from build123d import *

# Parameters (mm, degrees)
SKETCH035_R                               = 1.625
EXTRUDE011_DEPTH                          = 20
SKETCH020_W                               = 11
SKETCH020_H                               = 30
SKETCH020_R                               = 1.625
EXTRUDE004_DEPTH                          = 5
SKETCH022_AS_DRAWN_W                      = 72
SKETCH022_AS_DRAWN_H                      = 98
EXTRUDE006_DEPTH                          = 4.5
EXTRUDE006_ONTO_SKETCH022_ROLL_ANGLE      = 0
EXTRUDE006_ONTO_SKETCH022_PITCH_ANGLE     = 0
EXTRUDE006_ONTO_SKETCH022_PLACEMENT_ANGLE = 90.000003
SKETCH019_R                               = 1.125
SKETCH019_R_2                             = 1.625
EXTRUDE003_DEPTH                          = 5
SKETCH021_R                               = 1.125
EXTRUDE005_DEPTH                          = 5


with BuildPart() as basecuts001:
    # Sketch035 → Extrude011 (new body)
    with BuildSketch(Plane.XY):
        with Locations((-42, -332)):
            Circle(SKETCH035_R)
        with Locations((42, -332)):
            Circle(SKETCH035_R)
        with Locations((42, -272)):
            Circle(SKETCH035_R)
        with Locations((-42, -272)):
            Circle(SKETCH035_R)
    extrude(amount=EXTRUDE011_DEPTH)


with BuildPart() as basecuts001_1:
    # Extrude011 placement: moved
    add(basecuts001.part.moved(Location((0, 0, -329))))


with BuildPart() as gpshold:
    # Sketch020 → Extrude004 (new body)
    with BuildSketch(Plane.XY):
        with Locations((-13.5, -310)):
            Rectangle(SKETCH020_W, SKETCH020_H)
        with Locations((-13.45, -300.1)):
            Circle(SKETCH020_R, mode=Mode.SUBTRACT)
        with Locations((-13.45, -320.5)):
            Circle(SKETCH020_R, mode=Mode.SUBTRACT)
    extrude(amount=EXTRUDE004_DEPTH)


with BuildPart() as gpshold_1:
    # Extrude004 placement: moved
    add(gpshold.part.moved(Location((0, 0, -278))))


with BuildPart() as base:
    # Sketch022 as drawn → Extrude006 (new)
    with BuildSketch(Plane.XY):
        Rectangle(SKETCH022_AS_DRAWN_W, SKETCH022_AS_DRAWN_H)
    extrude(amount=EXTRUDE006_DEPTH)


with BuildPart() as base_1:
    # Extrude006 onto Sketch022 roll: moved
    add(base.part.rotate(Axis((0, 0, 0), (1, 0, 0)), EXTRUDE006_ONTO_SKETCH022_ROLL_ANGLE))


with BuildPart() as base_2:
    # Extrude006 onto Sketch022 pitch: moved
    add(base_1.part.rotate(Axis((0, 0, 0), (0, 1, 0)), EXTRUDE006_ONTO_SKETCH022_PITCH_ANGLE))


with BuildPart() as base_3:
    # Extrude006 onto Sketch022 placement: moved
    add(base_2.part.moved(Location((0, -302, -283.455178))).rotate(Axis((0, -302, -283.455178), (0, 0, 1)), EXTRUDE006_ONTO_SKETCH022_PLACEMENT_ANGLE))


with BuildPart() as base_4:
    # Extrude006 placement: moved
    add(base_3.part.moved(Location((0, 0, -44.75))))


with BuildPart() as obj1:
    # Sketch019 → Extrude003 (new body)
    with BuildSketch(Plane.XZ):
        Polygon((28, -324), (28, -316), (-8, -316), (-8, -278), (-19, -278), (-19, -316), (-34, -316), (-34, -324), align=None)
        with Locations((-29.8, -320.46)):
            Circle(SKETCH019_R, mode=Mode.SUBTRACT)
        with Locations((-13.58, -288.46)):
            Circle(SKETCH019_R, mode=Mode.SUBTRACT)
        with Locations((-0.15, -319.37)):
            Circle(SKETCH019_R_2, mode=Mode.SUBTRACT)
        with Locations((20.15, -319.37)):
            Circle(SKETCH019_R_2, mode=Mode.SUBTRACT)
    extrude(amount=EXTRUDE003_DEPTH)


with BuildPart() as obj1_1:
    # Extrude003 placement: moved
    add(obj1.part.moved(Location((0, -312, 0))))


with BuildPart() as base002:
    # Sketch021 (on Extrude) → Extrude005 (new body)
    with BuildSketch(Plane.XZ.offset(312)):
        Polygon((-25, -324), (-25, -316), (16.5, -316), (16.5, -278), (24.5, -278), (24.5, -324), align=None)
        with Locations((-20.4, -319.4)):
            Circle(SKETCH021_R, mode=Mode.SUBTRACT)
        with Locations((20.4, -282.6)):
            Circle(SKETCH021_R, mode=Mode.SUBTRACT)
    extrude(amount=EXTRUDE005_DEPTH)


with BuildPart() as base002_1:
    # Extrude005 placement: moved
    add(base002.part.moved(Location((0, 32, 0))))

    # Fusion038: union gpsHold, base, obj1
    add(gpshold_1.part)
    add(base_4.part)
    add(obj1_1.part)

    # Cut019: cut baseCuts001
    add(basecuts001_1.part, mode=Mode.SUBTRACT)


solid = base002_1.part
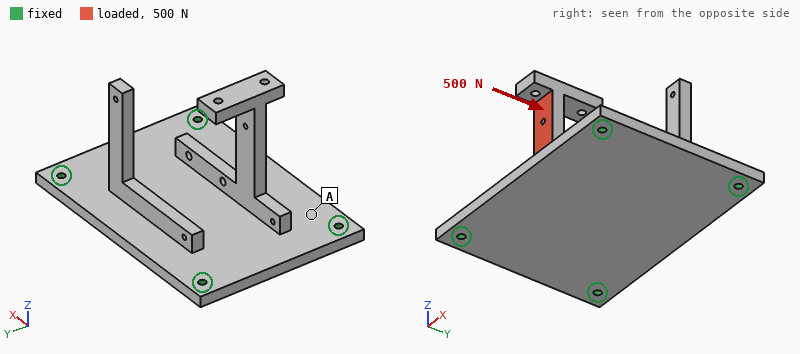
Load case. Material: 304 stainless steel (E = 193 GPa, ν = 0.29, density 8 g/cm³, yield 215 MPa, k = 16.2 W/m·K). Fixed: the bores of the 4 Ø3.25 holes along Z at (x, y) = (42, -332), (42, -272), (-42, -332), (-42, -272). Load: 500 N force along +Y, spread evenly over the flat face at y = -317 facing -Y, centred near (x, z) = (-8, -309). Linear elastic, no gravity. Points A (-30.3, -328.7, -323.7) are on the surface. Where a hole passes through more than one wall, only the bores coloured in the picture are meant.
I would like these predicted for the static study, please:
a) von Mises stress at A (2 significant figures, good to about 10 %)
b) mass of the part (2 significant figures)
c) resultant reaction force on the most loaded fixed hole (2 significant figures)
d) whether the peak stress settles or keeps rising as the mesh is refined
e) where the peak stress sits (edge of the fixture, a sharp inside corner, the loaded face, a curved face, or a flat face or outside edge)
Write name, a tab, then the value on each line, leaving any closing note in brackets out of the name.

von Mises stress at A	11 MPa
mass of the part	330 g
resultant reaction force on the most loaded fixed hole	210 N
whether the peak stress settles or keeps rising as the mesh is refined	keeps rising
where the peak stress sits	a sharp inside corner
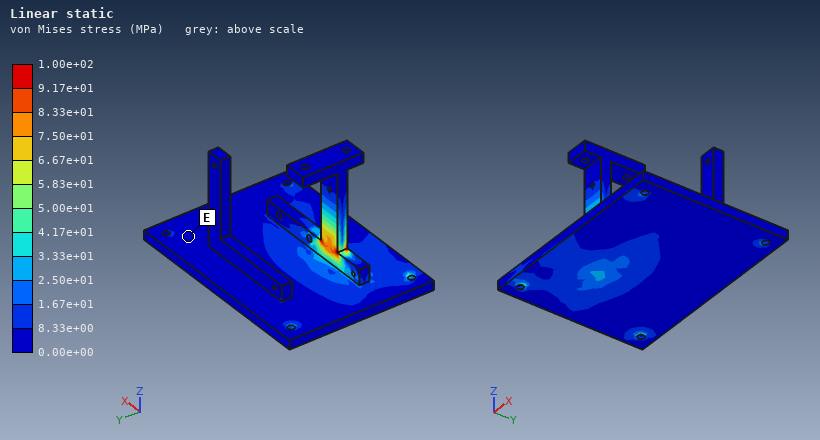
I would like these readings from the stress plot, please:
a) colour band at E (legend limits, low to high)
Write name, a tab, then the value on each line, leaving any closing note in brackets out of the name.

colour band at E	0.00e+00 to 8.33e+00 MPa
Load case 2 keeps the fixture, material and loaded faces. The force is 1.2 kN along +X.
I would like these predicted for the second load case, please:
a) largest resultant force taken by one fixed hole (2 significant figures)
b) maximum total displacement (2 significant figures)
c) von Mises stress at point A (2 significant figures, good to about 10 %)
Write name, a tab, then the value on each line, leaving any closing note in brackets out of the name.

largest resultant force taken by one fixed hole	470 N
maximum total displacement	0.10 mm
von Mises stress at point A	15 MPa
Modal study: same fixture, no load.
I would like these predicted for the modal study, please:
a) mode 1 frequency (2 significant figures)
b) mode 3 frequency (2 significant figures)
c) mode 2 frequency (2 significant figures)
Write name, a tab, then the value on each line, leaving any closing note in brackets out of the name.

mode 1 frequency	910 Hz
mode 3 frequency	2000 Hz
mode 2 frequency	1800 Hz
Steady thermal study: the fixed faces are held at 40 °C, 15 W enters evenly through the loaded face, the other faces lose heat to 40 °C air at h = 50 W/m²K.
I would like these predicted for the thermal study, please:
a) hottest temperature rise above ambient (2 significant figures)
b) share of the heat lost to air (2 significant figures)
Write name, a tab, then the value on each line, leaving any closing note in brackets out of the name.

hottest temperature rise above ambient	73 K
share of the heat lost to air	82 %
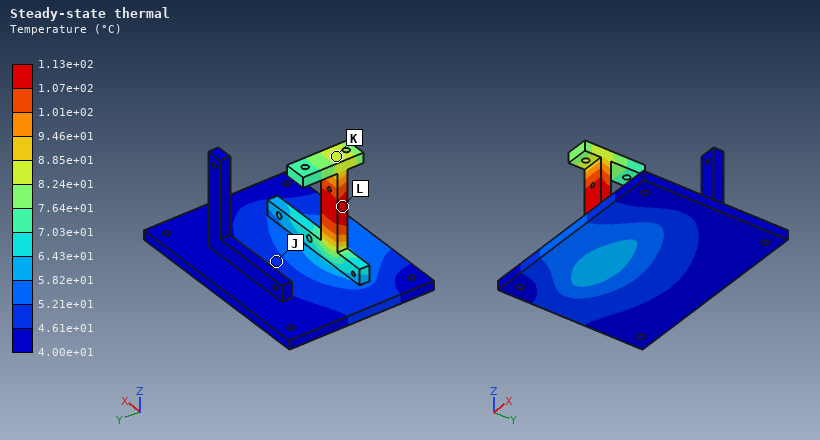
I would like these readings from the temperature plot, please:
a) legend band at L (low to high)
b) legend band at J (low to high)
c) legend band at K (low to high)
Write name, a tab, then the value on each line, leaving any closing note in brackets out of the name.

legend band at L	1.07e+02 to 1.13e+02 °C
legend band at J	4.61e+01 to 5.21e+01 °C
legend band at K	8.24e+01 to 8.85e+01 °C
